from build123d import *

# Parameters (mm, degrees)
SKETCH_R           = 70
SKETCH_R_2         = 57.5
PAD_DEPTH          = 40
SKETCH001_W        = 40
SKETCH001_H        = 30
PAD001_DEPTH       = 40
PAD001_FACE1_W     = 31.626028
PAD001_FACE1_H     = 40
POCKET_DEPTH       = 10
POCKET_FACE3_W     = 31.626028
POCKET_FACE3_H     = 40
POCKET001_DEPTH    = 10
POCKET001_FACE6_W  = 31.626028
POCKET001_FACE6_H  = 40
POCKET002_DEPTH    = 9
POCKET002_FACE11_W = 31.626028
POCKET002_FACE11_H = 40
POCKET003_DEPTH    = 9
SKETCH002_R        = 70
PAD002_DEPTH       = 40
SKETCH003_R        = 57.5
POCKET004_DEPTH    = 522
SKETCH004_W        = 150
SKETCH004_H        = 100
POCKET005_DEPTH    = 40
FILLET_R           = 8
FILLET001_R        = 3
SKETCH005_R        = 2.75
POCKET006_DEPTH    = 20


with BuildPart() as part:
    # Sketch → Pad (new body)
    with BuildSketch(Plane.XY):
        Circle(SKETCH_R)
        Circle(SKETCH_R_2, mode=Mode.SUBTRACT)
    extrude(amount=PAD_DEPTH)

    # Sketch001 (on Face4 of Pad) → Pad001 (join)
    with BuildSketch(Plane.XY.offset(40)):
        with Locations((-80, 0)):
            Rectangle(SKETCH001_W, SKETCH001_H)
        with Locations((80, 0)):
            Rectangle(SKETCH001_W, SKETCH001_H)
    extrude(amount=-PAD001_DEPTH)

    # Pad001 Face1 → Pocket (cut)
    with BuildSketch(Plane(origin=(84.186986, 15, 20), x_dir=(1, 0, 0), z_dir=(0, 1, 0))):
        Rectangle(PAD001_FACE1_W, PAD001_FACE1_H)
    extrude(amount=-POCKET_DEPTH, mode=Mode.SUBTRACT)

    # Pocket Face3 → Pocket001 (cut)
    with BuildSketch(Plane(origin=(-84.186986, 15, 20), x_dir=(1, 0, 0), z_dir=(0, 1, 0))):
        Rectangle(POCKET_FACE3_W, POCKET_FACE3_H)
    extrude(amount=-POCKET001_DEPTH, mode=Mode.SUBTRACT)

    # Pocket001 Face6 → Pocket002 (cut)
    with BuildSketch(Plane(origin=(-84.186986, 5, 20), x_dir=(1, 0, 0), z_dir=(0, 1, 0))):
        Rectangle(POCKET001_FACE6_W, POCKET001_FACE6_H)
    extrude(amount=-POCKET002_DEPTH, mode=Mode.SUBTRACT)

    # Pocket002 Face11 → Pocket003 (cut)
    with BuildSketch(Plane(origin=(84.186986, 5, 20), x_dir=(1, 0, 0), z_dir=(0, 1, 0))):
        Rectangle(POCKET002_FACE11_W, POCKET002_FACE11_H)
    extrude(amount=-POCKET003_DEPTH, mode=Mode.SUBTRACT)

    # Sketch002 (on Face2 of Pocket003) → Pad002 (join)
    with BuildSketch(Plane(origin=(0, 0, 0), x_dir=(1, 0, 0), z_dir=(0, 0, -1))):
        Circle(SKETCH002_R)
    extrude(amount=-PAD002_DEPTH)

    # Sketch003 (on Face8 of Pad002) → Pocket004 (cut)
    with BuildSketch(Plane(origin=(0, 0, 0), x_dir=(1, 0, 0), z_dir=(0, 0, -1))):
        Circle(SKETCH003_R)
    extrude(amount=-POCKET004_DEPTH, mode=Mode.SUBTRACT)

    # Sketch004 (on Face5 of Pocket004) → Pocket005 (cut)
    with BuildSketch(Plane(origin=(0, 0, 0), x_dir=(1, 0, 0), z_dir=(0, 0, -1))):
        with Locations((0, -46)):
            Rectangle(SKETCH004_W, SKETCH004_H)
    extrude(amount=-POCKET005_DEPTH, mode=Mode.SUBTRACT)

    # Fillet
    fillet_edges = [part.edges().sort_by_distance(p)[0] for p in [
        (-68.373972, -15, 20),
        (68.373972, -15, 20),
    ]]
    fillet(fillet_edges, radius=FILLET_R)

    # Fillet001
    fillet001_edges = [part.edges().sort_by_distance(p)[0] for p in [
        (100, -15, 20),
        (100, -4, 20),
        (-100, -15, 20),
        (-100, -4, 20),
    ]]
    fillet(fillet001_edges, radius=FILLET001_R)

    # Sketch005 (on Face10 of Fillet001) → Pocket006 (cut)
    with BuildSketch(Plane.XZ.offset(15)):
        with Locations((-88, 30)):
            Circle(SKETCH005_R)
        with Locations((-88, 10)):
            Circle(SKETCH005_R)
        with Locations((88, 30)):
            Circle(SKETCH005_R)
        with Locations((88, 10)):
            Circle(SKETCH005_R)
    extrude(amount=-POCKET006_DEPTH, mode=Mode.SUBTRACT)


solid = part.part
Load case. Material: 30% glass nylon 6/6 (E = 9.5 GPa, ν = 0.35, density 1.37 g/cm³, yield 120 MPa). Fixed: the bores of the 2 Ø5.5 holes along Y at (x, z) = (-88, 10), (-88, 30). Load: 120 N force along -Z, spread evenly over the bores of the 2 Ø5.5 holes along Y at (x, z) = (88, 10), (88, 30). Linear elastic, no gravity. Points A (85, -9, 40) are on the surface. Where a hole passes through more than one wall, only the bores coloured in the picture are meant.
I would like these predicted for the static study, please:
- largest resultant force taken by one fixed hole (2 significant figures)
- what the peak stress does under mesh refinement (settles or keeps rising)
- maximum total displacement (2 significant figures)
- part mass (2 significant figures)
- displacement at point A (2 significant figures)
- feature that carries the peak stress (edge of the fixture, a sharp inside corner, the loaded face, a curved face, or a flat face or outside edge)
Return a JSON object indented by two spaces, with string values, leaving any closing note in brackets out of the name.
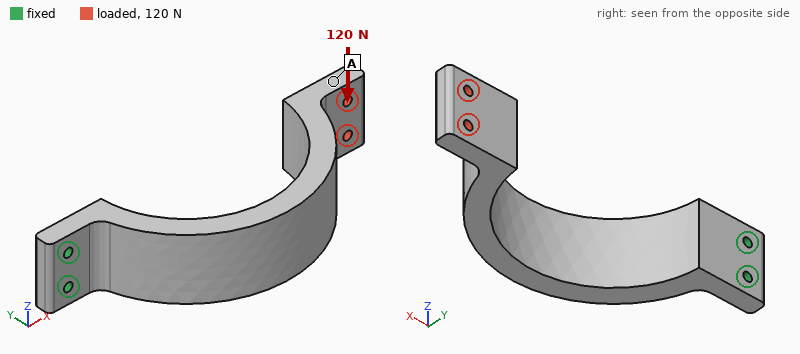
{
  "largest resultant force taken by one fixed hole": "910 N",
  "what the peak stress does under mesh refinement": "keeps rising",
  "maximum total displacement": "2.3 mm",
  "part mass": "170 g",
  "displacement at point A": "2.0 mm",
  "feature that carries the peak stress": "edge of the fixture"
}
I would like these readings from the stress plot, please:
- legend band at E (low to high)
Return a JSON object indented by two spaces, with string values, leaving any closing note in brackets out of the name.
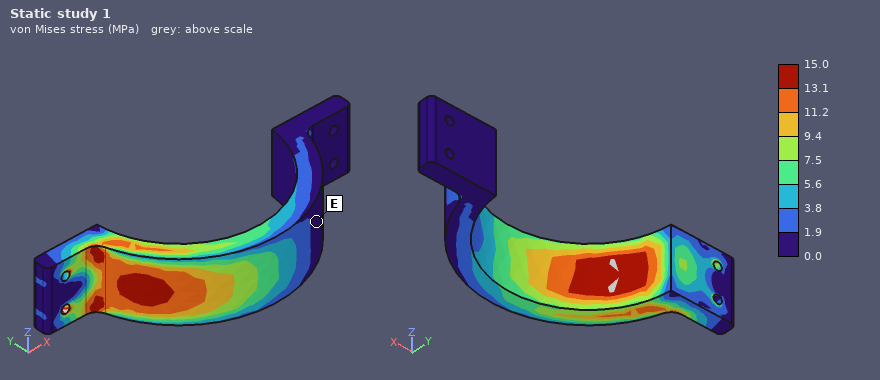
{
  "legend band at E": "0.0 to 1.9 MPa"
}
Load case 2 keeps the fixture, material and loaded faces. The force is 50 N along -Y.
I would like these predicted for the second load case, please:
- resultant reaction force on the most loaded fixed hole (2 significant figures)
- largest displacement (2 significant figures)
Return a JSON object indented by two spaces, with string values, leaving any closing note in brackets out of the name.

{
  "resultant reaction force on the most loaded fixed hole": "34 N",
  "largest displacement": "2.3 mm"
}
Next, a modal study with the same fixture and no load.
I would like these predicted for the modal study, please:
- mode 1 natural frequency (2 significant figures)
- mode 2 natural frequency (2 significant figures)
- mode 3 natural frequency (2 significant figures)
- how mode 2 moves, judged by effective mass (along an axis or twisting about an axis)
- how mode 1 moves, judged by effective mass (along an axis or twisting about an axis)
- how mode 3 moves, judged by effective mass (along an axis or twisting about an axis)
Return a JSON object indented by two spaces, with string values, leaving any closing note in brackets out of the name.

{
  "mode 1 natural frequency": "110 Hz",
  "mode 2 natural frequency": "190 Hz",
  "mode 3 natural frequency": "380 Hz",
  "how mode 2 moves, judged by effective mass": "along Z",
  "how mode 1 moves, judged by effective mass": "along Y",
  "how mode 3 moves, judged by effective mass": "along X"
}
